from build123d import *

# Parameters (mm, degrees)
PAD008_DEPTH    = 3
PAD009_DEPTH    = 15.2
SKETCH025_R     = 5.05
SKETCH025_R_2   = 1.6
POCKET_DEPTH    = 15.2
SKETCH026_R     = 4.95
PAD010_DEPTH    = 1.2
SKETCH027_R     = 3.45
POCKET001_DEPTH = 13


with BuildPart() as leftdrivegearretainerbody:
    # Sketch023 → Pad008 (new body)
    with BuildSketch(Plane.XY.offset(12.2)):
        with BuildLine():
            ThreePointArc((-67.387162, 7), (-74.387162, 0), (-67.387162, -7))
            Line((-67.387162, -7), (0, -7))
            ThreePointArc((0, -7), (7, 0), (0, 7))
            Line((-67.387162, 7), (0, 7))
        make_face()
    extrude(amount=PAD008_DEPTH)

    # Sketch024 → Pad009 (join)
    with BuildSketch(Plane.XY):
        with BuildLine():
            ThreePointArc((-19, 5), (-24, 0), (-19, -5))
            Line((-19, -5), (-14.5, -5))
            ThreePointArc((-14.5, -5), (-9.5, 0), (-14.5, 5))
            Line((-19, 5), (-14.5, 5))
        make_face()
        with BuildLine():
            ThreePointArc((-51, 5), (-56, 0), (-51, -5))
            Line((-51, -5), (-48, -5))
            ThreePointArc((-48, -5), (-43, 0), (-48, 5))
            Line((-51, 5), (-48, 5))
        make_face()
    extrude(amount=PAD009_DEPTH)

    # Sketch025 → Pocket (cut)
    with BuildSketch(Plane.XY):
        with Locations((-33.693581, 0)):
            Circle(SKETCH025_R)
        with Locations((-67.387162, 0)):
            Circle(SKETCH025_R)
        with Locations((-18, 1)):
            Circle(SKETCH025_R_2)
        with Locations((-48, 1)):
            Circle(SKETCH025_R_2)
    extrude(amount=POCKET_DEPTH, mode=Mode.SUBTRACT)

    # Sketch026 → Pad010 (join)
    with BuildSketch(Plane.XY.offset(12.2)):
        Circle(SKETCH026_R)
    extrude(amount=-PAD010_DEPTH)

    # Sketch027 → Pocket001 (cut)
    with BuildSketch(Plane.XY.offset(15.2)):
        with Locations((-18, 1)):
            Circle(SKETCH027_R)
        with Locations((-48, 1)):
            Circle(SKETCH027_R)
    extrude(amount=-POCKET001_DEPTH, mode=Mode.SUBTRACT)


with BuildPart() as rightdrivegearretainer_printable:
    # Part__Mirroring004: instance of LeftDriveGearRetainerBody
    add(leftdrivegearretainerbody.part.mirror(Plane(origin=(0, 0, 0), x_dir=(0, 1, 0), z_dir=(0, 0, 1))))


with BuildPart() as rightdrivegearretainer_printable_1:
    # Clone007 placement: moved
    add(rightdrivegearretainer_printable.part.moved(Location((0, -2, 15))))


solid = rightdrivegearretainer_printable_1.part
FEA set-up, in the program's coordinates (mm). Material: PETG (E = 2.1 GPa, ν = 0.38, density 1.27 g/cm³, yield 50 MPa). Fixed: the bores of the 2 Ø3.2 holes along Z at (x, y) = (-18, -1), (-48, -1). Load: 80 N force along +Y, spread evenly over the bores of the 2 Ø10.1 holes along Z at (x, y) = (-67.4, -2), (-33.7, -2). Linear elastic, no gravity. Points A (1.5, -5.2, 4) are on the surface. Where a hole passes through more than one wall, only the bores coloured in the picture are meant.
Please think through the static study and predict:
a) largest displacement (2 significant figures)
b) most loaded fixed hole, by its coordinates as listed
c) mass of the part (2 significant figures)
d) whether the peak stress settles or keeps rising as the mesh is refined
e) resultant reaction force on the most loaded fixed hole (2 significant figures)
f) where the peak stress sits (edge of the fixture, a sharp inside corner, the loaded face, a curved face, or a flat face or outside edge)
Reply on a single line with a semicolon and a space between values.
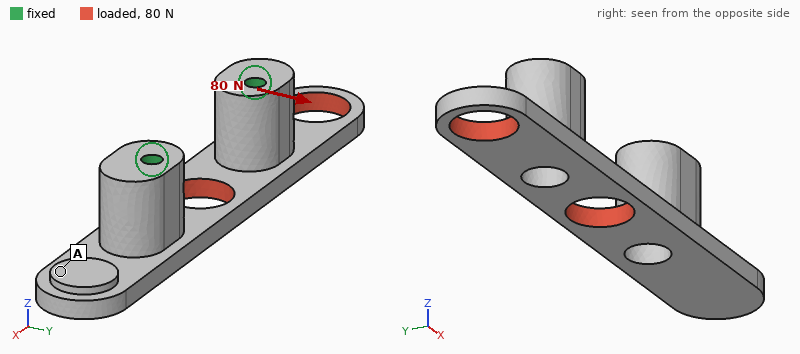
0.89 mm; (-48, -1); 6.0 g; keeps rising; 64 N; edge of the fixture
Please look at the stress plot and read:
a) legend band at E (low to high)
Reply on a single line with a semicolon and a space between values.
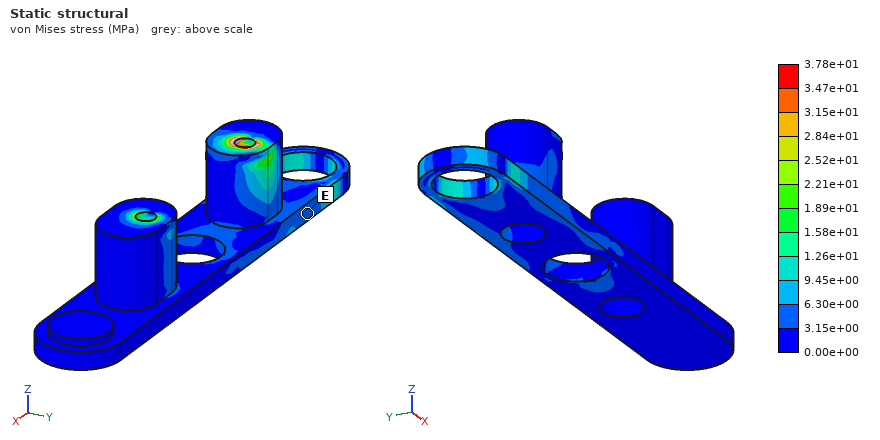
3.15e+00 to 6.30e+00 MPa
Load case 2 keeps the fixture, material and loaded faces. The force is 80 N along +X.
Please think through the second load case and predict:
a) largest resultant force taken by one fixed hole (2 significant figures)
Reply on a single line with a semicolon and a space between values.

42 N
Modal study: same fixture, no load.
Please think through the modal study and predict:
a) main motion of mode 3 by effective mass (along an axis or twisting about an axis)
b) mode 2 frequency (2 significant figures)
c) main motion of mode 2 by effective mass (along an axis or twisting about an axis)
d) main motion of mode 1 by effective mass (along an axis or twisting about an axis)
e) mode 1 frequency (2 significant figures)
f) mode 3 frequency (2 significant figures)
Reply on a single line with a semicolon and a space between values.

along Y; 1300 Hz; along Y; along X; 1200 Hz; 1500 Hz
